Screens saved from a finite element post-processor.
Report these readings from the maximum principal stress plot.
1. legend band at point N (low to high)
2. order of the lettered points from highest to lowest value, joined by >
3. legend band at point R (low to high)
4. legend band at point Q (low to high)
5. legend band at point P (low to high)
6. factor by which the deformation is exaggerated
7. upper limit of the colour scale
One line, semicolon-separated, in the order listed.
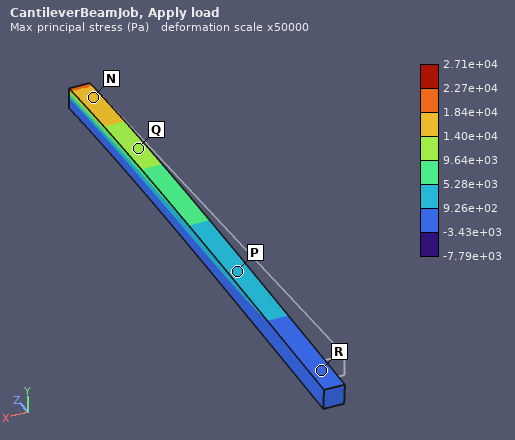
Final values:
1.40e+04 to 1.84e+04 Pa; N > Q > P > R; -3.43e+03 to 9.26e+02 Pa; 9.64e+03 to 1.40e+04 Pa; 9.26e+02 to 5.28e+03 Pa; 50000; 2.71e+04 Pa
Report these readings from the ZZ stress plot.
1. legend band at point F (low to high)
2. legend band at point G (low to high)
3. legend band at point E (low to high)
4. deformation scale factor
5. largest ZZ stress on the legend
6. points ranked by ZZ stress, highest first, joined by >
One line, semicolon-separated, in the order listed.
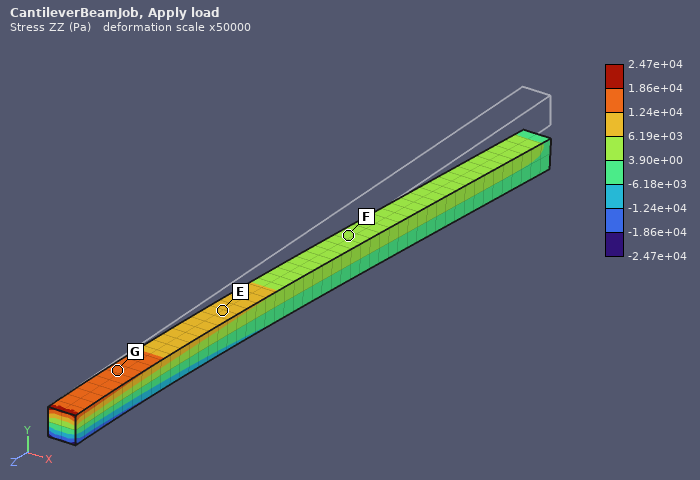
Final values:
3.90e+00 to 6.19e+03 Pa; 1.24e+04 to 1.86e+04 Pa; 6.19e+03 to 1.24e+04 Pa; 50000; 2.47e+04 Pa; G > E > F
